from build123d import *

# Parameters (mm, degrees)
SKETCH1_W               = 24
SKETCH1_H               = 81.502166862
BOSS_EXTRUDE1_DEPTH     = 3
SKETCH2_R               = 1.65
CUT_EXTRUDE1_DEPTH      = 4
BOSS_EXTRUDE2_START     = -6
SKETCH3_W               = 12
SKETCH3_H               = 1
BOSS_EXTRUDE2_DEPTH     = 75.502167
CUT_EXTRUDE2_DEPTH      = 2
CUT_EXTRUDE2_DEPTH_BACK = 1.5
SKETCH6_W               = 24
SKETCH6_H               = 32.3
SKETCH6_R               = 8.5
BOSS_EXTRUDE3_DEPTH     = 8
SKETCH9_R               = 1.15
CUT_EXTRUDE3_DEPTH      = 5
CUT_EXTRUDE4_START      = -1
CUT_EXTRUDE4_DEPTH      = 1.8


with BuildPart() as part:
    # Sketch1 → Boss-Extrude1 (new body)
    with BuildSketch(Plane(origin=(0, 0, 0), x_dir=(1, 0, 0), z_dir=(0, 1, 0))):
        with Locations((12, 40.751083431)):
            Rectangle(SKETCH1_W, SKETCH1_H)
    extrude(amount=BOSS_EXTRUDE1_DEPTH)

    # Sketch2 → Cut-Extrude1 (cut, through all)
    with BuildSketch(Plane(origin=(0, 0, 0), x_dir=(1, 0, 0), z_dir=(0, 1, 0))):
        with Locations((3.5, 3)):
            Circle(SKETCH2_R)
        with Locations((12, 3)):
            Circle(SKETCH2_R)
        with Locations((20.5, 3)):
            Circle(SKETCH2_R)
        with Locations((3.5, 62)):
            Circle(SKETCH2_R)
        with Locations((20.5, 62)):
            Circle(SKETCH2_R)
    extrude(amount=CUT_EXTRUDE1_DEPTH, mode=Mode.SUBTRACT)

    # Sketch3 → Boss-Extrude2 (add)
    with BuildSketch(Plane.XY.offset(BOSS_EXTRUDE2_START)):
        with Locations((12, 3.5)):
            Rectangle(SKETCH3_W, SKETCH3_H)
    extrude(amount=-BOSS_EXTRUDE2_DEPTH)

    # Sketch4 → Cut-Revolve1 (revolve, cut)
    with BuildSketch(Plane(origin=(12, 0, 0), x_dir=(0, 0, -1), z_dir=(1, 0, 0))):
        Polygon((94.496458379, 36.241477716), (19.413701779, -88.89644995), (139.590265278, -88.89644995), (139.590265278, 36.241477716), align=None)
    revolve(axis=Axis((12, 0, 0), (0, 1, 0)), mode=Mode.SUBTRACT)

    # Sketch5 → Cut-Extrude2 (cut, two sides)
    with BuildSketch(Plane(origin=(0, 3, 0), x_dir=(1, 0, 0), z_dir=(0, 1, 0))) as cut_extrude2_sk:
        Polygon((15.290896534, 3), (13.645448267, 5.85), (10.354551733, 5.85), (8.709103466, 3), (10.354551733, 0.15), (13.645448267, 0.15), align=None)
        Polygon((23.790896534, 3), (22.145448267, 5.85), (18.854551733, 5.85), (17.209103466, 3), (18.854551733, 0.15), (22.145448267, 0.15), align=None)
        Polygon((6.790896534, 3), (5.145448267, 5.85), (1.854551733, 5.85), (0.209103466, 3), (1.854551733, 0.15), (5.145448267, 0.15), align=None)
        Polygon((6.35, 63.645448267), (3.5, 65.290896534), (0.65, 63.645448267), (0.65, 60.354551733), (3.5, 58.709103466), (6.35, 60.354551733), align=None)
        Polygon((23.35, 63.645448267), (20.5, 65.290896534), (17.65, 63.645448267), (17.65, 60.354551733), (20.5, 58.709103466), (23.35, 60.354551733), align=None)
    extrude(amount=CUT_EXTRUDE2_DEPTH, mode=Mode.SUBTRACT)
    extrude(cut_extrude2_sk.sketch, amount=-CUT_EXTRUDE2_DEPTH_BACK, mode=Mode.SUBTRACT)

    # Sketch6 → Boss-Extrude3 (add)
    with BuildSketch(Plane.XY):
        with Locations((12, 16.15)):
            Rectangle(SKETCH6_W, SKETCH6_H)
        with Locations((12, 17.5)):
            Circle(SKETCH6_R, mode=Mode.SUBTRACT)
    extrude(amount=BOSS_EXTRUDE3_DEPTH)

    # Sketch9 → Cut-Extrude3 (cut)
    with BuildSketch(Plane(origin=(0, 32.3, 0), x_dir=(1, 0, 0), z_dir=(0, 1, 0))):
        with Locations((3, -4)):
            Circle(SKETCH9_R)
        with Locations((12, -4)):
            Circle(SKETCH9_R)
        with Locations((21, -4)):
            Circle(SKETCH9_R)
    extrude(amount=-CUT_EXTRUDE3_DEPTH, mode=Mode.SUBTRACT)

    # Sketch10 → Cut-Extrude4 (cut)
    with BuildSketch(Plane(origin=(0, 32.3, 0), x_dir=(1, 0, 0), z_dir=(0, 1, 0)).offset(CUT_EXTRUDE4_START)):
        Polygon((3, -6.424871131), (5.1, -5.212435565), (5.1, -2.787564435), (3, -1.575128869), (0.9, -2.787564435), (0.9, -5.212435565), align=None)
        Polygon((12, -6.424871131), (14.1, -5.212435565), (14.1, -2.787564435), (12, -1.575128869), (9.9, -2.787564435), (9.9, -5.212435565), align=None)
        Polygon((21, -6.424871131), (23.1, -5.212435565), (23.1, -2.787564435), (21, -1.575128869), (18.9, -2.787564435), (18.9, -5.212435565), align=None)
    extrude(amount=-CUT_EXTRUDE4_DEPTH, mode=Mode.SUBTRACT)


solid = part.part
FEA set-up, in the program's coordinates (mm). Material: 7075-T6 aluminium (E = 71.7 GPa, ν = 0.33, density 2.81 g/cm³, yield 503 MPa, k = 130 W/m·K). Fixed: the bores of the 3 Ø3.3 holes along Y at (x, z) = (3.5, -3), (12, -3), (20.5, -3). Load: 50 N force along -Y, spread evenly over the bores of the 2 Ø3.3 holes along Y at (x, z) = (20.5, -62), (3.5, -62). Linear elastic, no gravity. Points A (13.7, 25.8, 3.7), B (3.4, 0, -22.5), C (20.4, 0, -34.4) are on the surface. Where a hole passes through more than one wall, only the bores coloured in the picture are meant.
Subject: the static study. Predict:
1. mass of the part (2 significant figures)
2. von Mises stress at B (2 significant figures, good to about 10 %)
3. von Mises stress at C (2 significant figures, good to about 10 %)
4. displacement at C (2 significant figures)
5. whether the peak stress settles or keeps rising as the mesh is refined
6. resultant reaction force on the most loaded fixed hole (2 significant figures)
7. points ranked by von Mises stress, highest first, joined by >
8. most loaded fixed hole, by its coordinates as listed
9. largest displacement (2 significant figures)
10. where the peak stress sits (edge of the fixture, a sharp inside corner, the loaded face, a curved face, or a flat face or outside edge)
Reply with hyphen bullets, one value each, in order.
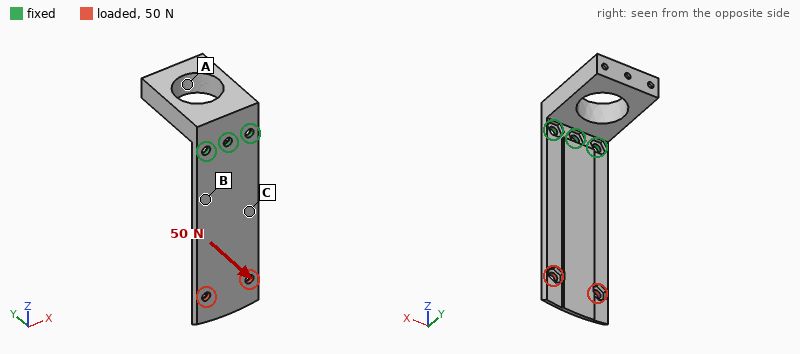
- 28 g
- 37 MPa
- 26 MPa
- 0.29 mm
- keeps rising
- 64 N
- B > C > A
- (12, -3)
- 0.94 mm
- edge of the fixture
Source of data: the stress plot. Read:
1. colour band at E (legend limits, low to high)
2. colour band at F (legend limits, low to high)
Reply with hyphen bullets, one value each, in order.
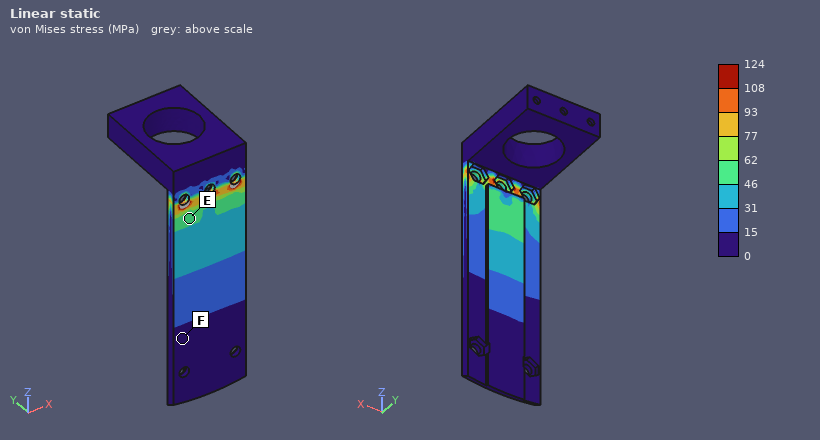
- 46 to 62 MPa
- 0 to 15 MPa
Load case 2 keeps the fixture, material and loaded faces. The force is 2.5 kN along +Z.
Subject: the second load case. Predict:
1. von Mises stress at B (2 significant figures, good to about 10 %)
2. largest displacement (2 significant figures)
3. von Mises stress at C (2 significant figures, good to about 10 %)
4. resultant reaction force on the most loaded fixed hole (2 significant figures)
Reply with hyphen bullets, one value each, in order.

- 78 MPa
- 0.90 mm
- 78 MPa
- 850 N
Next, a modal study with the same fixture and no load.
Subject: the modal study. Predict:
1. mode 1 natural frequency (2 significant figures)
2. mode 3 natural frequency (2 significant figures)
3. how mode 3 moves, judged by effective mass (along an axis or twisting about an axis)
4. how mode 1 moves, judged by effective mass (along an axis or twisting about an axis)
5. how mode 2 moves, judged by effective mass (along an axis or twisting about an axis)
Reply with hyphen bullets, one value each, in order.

- 510 Hz
- 3100 Hz
- along X
- along Y
- along Z
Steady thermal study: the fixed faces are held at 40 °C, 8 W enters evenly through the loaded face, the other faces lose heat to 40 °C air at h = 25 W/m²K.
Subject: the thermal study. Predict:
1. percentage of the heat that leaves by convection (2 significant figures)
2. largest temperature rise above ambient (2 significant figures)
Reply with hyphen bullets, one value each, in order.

- 27 %
- 40 K
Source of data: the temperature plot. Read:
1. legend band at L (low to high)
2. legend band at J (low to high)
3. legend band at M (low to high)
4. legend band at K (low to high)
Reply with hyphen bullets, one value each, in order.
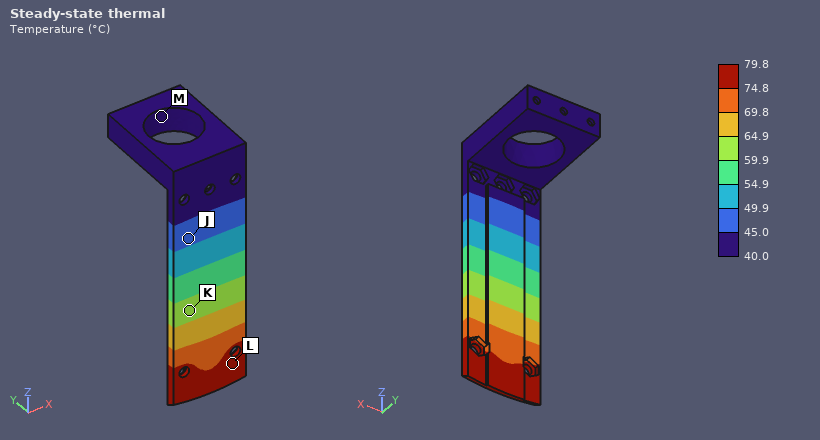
- 74.8 to 79.8 °C
- 45.0 to 49.9 °C
- 40.0 to 45.0 °C
- 59.9 to 64.9 °C
